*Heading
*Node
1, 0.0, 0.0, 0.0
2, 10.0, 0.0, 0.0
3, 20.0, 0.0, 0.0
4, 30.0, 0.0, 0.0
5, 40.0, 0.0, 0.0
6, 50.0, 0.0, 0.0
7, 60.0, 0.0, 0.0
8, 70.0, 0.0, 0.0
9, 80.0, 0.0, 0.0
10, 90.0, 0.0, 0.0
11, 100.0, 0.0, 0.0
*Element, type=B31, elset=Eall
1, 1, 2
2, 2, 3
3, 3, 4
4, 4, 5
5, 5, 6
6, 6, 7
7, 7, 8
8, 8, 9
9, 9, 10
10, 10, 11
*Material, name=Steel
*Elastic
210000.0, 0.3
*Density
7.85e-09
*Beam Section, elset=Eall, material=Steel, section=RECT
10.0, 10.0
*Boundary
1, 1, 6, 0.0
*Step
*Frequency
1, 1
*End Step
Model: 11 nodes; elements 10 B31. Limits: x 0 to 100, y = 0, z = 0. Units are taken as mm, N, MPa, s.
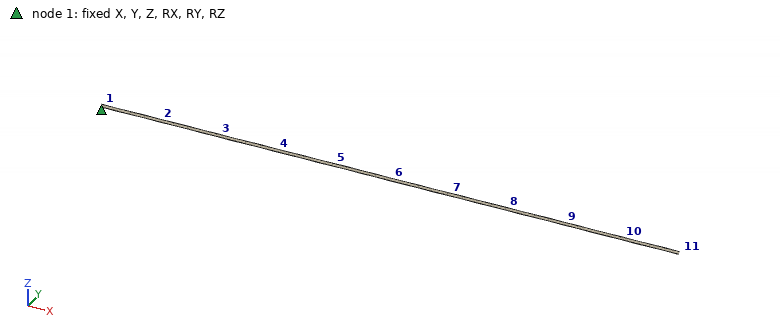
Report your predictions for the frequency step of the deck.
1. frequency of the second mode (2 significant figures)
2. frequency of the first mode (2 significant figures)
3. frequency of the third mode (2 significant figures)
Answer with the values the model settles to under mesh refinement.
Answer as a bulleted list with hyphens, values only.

- 830 Hz
- 830 Hz
- 5000 Hz
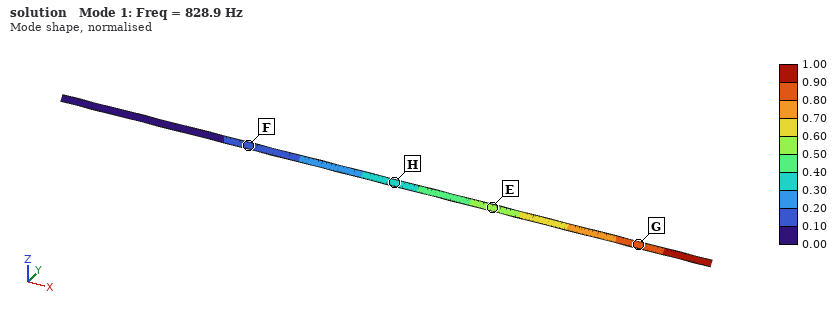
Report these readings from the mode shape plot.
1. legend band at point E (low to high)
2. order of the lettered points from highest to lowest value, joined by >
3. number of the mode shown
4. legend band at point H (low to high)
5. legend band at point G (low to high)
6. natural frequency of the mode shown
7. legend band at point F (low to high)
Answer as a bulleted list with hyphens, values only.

- 0.50 to 0.60
- G > E > H > F
- 1
- 0.30 to 0.40
- 0.80 to 0.90
- 828.9 Hz
- 0.10 to 0.20
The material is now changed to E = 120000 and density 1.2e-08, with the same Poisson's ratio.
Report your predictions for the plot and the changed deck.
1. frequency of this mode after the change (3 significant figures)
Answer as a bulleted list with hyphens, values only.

- 507 Hz
